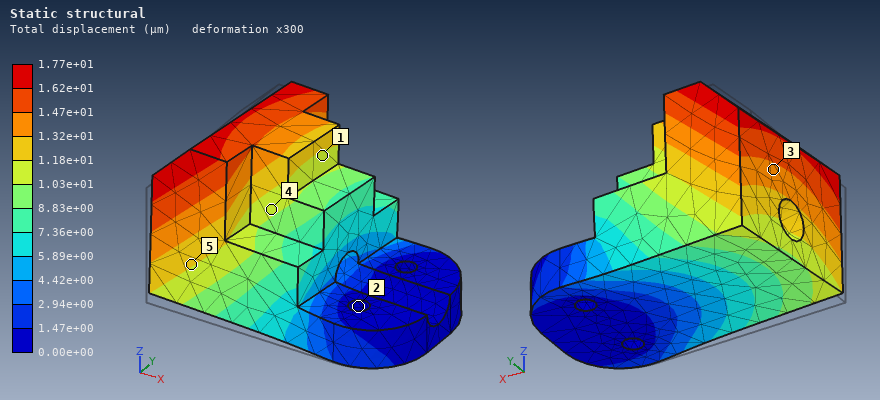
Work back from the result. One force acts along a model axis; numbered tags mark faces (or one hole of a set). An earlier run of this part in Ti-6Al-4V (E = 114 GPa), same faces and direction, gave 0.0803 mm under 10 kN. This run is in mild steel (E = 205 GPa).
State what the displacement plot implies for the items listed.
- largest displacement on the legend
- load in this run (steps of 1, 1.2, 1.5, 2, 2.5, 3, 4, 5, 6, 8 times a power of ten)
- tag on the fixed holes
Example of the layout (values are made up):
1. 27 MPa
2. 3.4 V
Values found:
1. 1.77e+01 µm
2. 4 kN
3. 2
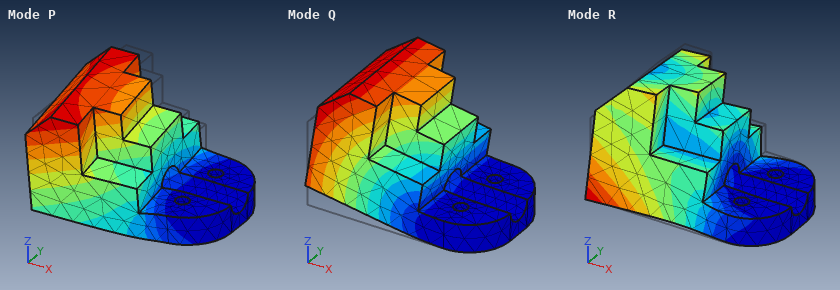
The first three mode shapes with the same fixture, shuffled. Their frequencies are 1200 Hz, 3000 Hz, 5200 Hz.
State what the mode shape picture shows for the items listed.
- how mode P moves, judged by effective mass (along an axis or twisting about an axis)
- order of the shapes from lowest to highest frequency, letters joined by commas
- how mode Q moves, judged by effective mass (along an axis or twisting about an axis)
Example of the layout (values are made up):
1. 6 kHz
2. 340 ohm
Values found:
1. along Y
2. Q, P, R
3. along Z
